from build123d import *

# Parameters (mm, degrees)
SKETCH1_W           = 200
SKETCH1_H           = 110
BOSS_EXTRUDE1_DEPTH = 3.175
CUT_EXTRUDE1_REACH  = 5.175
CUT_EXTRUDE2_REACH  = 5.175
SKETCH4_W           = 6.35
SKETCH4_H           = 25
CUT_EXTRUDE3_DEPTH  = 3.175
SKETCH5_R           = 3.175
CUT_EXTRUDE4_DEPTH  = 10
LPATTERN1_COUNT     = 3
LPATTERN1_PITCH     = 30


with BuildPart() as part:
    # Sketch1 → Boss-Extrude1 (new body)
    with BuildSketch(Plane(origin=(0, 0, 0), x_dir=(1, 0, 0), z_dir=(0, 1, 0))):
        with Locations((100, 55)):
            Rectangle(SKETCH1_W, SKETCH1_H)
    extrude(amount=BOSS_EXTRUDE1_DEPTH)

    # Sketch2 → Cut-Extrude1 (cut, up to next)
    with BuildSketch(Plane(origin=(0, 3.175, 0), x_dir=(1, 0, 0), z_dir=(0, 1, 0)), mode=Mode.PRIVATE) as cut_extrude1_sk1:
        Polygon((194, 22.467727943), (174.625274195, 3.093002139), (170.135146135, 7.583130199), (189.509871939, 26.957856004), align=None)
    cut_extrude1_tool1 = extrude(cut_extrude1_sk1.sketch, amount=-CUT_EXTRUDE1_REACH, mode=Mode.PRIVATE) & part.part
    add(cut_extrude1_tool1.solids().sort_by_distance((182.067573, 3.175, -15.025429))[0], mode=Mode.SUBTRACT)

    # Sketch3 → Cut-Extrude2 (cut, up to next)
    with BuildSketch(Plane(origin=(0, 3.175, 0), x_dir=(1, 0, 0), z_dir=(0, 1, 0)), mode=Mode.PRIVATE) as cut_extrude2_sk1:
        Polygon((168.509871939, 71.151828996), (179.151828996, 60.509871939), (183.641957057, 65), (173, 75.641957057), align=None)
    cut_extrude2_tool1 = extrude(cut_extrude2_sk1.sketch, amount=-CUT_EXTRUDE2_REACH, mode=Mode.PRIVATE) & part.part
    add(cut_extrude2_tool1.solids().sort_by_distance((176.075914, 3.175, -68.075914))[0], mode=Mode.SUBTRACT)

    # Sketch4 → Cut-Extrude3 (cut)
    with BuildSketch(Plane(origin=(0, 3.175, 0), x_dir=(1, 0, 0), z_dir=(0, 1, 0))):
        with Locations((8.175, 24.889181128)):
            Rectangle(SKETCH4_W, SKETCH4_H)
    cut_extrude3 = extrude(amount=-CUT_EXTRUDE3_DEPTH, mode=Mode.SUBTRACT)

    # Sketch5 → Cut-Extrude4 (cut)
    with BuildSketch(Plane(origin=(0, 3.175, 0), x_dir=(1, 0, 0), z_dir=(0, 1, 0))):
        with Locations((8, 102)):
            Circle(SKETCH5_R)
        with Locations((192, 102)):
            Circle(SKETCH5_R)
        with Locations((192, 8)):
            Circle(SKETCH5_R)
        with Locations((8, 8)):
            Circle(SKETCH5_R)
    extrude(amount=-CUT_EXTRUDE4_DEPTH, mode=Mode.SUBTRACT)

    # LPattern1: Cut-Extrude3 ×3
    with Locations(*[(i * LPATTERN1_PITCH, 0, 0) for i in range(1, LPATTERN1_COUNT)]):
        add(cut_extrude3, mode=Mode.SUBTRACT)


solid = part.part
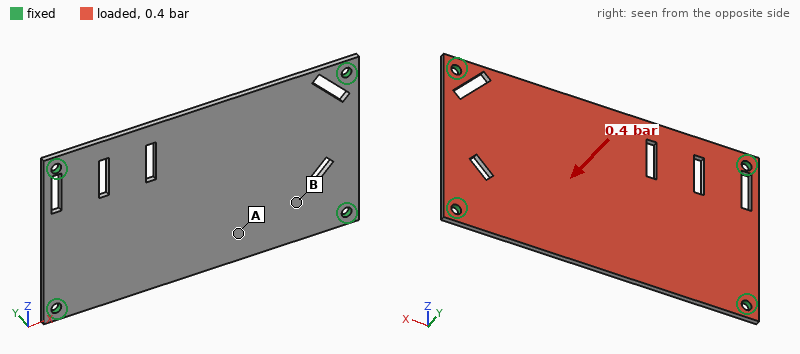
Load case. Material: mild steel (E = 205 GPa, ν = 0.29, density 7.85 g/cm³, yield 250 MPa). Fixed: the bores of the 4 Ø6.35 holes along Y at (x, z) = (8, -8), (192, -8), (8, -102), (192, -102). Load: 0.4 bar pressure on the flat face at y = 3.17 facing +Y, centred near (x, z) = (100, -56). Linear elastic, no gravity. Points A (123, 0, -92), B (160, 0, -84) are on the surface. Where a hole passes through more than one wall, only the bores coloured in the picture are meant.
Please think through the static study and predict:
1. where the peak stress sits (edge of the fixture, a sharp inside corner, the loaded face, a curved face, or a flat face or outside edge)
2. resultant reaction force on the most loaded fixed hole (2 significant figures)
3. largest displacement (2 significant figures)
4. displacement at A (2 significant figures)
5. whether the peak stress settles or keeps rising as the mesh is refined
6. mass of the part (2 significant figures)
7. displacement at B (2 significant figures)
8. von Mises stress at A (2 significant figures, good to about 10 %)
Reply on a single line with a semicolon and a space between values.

edge of the fixture; 240 N; 0.35 mm; 0.28 mm; keeps rising; 530 g; 0.13 mm; 35 MPa
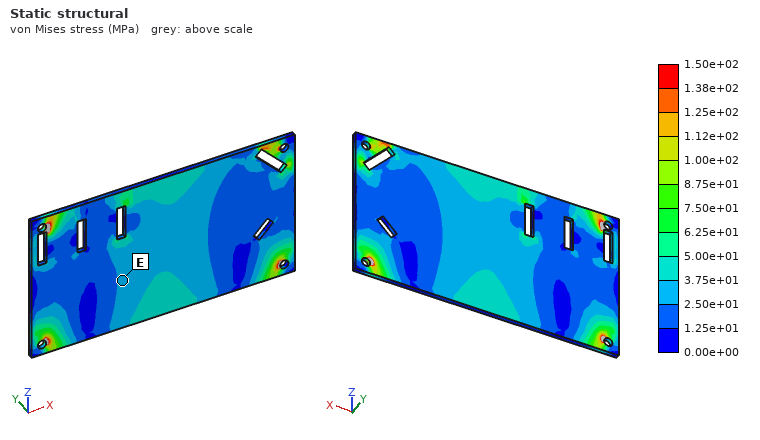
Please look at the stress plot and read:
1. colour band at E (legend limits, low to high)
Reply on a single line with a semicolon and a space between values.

2.50e+01 to 3.75e+01 MPa
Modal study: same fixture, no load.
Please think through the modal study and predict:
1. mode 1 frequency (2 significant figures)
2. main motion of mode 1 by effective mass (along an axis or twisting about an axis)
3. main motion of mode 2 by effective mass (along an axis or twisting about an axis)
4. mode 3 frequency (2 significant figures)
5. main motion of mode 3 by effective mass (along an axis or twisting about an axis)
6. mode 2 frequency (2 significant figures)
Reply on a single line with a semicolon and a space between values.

400 Hz; along Y; twisting about X; 1100 Hz; twisting about Z; 720 Hz
